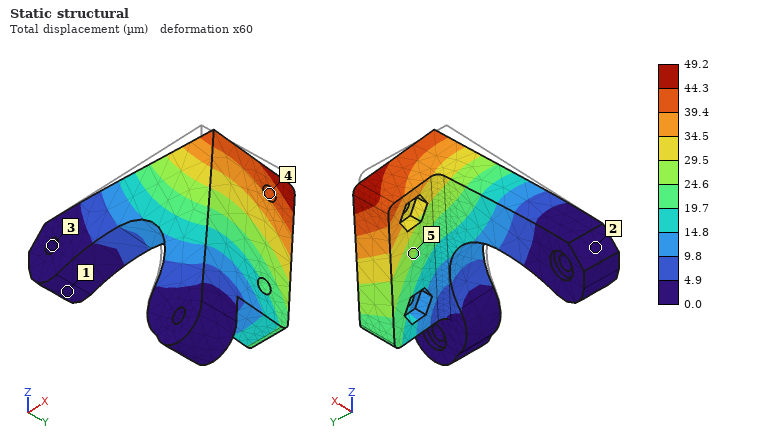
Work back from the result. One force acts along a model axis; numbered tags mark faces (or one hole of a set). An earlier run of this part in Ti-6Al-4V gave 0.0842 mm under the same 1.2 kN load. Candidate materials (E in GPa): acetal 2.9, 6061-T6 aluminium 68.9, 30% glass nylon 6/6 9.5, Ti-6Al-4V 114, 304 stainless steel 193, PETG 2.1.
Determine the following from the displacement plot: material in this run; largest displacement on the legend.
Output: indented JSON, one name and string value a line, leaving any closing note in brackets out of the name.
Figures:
{
  "material in this run": "304 stainless steel",
  "largest displacement on the legend": "49.2 µm"
}
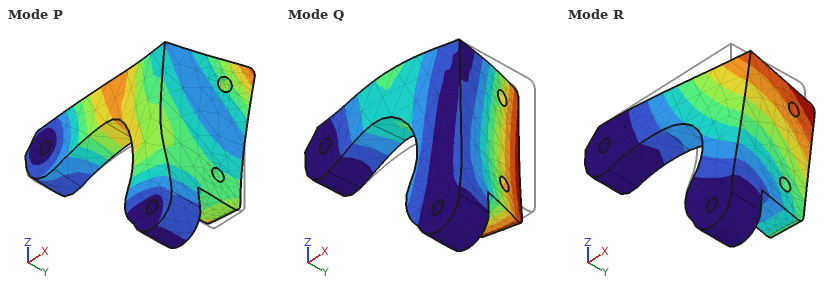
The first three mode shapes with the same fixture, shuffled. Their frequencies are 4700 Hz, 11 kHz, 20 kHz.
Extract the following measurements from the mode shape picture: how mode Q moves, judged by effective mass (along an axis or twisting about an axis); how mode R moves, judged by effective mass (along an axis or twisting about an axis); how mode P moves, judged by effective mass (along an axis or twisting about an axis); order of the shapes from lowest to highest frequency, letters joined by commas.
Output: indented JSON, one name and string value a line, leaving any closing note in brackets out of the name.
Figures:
{
  "how mode Q moves, judged by effective mass": "along X",
  "how mode R moves, judged by effective mass": "along Y",
  "how mode P moves, judged by effective mass": "along Z",
  "order of the shapes from lowest to highest frequency, letters joined by commas": "R, Q, P"
}
